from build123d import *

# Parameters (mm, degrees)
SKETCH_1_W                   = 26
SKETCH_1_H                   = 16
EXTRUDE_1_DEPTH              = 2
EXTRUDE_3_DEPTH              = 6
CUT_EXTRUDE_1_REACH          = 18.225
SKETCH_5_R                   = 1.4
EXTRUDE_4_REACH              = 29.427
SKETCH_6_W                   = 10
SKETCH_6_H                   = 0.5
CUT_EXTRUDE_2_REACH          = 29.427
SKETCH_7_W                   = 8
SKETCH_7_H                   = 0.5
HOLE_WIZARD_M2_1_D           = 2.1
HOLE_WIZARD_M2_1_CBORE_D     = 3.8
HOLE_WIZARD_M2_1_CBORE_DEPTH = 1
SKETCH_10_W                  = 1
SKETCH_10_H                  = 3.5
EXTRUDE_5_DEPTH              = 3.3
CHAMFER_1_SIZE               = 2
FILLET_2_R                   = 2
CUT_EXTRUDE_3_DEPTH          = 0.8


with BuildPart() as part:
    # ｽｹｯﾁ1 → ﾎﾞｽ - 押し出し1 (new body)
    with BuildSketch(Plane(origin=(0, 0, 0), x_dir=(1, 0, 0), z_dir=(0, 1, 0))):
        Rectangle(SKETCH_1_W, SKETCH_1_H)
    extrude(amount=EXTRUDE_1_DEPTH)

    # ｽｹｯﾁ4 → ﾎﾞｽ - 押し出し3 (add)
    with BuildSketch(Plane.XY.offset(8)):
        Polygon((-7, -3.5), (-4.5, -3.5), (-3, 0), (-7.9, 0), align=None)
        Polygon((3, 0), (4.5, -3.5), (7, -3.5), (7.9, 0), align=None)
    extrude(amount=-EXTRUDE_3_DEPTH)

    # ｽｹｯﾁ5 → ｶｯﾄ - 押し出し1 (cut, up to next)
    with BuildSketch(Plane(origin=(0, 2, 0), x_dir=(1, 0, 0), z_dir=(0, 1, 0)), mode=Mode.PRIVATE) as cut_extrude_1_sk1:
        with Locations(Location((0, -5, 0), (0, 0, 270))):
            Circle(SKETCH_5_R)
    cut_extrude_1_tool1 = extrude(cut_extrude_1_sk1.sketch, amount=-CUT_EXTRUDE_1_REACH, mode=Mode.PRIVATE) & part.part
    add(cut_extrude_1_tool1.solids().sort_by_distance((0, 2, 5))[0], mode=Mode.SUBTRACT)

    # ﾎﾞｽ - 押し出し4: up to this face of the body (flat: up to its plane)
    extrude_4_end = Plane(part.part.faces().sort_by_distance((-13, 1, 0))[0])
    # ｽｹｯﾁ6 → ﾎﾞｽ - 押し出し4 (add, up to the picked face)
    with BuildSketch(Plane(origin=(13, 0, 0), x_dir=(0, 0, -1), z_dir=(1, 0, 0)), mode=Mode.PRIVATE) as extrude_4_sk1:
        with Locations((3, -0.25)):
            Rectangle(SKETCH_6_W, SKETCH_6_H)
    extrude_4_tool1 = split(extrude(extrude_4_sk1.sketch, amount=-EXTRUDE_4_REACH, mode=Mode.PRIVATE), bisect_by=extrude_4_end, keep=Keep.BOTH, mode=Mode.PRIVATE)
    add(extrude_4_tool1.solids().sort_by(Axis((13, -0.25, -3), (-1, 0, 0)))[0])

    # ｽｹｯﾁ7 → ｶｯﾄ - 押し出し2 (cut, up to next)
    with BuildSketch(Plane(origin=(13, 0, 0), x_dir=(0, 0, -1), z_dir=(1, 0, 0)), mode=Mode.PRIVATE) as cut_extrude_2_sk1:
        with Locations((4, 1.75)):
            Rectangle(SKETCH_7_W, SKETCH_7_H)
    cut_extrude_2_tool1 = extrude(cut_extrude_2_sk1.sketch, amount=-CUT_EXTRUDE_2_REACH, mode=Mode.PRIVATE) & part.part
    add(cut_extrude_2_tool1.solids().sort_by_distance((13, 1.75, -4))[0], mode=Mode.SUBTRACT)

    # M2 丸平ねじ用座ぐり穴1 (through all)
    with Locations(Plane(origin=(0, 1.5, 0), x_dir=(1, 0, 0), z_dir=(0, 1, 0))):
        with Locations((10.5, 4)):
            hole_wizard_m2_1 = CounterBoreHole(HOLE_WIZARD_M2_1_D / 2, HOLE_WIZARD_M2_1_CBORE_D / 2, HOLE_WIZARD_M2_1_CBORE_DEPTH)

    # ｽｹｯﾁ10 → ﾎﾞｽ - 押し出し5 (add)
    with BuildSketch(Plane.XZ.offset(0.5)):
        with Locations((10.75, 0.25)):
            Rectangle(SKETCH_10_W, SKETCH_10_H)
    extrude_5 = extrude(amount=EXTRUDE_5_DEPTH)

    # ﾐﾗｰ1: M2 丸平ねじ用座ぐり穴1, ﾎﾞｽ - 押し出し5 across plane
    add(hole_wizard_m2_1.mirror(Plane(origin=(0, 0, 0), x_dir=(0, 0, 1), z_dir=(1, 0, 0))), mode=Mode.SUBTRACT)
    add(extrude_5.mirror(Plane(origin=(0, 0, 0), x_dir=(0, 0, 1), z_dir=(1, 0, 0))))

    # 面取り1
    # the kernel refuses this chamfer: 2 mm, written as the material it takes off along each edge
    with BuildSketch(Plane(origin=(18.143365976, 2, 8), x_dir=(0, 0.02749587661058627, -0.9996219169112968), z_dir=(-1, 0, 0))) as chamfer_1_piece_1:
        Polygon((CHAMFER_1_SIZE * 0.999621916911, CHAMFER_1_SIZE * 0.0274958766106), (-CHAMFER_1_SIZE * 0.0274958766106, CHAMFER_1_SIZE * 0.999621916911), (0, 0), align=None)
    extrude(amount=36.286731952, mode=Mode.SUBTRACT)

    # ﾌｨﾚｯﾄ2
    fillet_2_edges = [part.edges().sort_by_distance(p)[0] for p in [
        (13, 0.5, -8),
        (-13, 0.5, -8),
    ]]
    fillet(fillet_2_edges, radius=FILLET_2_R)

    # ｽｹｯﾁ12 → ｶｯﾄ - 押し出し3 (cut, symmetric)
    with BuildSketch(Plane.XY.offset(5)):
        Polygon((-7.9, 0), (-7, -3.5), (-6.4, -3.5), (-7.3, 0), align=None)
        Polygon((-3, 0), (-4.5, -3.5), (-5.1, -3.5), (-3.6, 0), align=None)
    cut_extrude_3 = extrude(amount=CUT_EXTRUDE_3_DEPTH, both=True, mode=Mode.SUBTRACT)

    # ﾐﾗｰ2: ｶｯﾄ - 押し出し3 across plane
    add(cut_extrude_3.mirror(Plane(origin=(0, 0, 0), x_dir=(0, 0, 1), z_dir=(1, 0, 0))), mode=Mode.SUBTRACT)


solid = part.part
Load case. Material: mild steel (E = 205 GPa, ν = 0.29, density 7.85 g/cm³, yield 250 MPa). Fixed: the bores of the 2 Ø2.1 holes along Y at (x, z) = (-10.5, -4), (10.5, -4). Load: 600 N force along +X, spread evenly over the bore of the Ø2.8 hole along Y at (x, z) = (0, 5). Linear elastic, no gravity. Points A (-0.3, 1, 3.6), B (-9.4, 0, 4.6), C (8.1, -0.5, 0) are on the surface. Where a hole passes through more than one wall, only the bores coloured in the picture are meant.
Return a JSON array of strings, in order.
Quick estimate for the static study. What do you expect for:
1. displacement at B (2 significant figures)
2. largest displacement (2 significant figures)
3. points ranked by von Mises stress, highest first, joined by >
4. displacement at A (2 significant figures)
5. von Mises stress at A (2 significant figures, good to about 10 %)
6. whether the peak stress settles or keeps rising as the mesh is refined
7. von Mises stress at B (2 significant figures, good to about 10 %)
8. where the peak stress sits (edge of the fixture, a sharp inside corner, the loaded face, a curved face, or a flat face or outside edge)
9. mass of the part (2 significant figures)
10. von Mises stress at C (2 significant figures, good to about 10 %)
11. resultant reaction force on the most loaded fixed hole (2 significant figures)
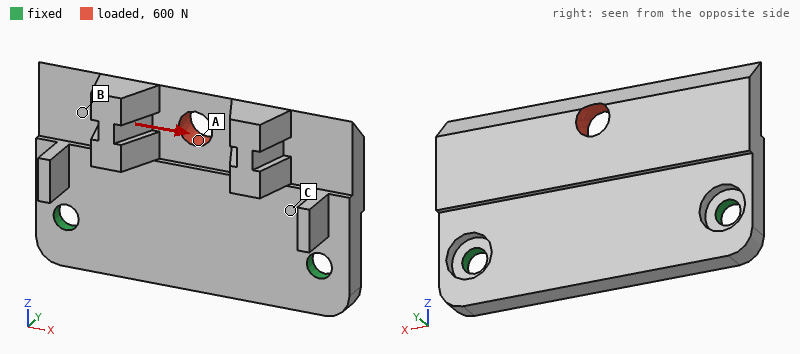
["2.3 µm", "3.4 µm", "A > C > B", "2.3 µm", "65 MPa", "keeps rising", "14 MPa", "edge of the fixture", "7.3 g", "35 MPa", "390 N"]
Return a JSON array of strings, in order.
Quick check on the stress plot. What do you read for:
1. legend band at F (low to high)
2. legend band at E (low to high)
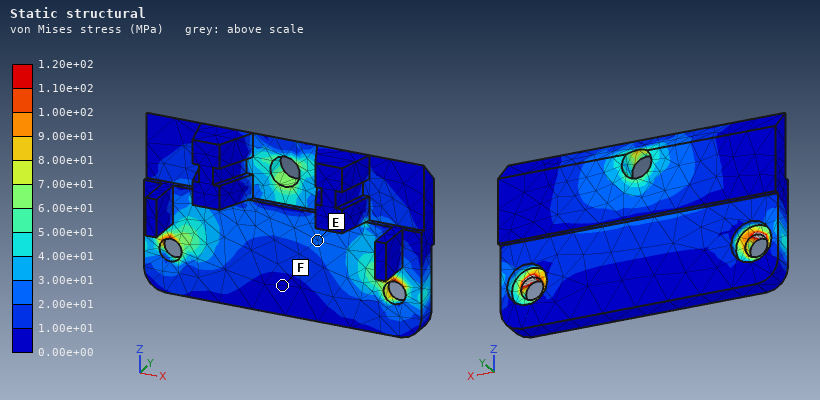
["0.00e+00 to 1.00e+01 MPa", "2.00e+01 to 3.00e+01 MPa"]
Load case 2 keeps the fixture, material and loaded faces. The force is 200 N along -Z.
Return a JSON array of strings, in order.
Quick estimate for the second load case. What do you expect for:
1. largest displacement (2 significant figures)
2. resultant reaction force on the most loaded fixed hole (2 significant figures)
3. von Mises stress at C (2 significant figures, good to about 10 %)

["6.2 µm", "110 N", "8.6 MPa"]
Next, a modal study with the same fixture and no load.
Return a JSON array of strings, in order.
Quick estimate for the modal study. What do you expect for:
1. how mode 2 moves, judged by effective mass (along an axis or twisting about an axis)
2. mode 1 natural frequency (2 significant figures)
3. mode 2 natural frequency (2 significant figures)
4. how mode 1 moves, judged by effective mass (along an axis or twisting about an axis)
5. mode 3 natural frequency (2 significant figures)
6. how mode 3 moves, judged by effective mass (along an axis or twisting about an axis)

["twisting about Z", "5900 Hz", "14 kHz", "along Y", "18 kHz", "along Y"]
